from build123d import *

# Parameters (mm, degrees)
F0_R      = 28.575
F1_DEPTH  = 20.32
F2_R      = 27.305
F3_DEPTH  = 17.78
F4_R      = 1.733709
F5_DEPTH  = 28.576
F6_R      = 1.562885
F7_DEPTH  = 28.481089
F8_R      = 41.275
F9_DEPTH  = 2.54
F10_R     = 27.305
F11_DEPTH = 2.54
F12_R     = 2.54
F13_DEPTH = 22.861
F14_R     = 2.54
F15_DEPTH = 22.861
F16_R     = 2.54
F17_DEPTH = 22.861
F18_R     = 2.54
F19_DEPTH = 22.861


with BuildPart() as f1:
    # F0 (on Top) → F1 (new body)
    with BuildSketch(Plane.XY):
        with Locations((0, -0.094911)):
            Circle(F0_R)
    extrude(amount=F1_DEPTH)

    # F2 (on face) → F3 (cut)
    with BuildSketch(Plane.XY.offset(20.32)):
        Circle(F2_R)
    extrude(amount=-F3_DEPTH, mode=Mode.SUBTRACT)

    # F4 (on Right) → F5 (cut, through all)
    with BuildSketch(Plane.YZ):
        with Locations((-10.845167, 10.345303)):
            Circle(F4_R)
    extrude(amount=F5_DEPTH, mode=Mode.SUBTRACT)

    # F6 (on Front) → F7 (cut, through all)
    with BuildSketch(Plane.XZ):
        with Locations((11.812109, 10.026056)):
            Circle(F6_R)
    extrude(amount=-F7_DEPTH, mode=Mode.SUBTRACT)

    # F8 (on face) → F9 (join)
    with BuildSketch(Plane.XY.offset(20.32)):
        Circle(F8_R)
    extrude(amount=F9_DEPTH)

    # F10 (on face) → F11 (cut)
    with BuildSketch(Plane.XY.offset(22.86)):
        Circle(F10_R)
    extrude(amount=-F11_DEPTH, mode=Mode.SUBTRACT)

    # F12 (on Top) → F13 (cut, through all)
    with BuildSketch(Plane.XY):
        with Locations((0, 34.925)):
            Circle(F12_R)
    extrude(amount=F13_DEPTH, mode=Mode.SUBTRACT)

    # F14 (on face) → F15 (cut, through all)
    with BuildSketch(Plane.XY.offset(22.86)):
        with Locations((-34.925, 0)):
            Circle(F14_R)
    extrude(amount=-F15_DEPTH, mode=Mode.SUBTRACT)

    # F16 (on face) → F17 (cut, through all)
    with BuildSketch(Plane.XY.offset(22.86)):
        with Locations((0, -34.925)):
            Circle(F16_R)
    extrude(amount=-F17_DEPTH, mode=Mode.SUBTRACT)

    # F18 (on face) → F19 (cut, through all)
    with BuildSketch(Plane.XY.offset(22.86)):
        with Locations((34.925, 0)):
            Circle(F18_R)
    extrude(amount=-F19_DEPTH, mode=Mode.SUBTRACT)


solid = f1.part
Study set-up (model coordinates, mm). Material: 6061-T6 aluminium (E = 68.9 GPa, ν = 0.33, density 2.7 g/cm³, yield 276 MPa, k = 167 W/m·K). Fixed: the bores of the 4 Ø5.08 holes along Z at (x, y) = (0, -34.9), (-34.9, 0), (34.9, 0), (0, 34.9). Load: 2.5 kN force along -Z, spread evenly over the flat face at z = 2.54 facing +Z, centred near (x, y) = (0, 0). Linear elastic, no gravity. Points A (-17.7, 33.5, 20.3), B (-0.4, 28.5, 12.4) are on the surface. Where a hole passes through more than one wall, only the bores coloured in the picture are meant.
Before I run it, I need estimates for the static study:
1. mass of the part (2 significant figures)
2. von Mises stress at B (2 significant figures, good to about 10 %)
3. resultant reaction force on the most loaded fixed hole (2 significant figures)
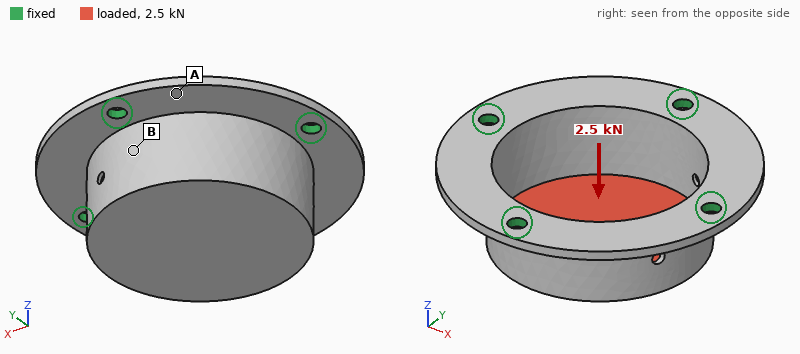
48 g
38 MPa
640 N
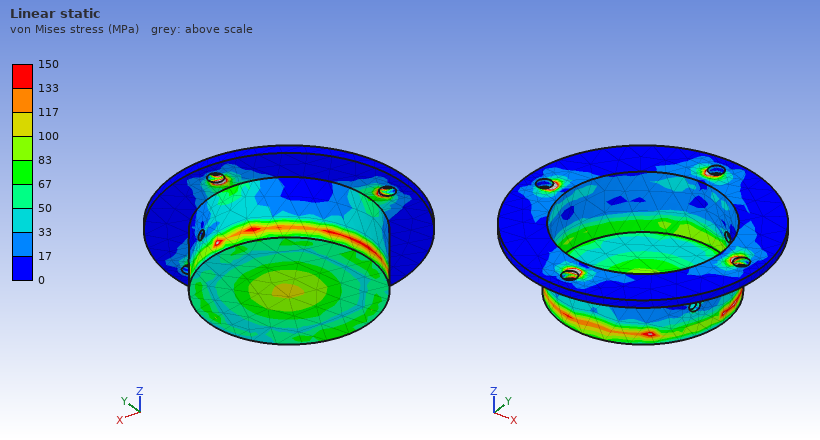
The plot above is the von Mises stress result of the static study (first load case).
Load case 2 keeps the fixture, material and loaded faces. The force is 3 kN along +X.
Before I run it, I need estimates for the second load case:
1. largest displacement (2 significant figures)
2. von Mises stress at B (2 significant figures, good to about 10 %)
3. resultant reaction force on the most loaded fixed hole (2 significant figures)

68 µm
39 MPa
1.1 kN
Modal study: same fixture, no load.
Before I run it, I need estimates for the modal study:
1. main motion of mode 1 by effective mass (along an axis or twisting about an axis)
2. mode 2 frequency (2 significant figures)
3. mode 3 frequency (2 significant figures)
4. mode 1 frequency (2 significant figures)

along Z
6200 Hz
6200 Hz
5100 Hz
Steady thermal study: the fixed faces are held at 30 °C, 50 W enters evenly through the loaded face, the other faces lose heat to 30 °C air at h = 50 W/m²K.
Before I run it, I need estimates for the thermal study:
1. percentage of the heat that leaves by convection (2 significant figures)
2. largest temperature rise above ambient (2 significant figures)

26 %
39 K
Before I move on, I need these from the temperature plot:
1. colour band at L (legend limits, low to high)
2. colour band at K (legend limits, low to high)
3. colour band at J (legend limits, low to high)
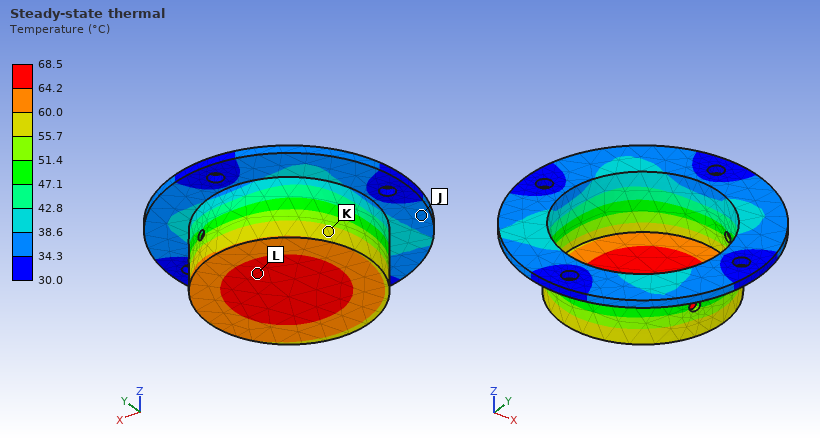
64.2 to 68.5 °C
55.7 to 60.0 °C
34.3 to 38.6 °C
